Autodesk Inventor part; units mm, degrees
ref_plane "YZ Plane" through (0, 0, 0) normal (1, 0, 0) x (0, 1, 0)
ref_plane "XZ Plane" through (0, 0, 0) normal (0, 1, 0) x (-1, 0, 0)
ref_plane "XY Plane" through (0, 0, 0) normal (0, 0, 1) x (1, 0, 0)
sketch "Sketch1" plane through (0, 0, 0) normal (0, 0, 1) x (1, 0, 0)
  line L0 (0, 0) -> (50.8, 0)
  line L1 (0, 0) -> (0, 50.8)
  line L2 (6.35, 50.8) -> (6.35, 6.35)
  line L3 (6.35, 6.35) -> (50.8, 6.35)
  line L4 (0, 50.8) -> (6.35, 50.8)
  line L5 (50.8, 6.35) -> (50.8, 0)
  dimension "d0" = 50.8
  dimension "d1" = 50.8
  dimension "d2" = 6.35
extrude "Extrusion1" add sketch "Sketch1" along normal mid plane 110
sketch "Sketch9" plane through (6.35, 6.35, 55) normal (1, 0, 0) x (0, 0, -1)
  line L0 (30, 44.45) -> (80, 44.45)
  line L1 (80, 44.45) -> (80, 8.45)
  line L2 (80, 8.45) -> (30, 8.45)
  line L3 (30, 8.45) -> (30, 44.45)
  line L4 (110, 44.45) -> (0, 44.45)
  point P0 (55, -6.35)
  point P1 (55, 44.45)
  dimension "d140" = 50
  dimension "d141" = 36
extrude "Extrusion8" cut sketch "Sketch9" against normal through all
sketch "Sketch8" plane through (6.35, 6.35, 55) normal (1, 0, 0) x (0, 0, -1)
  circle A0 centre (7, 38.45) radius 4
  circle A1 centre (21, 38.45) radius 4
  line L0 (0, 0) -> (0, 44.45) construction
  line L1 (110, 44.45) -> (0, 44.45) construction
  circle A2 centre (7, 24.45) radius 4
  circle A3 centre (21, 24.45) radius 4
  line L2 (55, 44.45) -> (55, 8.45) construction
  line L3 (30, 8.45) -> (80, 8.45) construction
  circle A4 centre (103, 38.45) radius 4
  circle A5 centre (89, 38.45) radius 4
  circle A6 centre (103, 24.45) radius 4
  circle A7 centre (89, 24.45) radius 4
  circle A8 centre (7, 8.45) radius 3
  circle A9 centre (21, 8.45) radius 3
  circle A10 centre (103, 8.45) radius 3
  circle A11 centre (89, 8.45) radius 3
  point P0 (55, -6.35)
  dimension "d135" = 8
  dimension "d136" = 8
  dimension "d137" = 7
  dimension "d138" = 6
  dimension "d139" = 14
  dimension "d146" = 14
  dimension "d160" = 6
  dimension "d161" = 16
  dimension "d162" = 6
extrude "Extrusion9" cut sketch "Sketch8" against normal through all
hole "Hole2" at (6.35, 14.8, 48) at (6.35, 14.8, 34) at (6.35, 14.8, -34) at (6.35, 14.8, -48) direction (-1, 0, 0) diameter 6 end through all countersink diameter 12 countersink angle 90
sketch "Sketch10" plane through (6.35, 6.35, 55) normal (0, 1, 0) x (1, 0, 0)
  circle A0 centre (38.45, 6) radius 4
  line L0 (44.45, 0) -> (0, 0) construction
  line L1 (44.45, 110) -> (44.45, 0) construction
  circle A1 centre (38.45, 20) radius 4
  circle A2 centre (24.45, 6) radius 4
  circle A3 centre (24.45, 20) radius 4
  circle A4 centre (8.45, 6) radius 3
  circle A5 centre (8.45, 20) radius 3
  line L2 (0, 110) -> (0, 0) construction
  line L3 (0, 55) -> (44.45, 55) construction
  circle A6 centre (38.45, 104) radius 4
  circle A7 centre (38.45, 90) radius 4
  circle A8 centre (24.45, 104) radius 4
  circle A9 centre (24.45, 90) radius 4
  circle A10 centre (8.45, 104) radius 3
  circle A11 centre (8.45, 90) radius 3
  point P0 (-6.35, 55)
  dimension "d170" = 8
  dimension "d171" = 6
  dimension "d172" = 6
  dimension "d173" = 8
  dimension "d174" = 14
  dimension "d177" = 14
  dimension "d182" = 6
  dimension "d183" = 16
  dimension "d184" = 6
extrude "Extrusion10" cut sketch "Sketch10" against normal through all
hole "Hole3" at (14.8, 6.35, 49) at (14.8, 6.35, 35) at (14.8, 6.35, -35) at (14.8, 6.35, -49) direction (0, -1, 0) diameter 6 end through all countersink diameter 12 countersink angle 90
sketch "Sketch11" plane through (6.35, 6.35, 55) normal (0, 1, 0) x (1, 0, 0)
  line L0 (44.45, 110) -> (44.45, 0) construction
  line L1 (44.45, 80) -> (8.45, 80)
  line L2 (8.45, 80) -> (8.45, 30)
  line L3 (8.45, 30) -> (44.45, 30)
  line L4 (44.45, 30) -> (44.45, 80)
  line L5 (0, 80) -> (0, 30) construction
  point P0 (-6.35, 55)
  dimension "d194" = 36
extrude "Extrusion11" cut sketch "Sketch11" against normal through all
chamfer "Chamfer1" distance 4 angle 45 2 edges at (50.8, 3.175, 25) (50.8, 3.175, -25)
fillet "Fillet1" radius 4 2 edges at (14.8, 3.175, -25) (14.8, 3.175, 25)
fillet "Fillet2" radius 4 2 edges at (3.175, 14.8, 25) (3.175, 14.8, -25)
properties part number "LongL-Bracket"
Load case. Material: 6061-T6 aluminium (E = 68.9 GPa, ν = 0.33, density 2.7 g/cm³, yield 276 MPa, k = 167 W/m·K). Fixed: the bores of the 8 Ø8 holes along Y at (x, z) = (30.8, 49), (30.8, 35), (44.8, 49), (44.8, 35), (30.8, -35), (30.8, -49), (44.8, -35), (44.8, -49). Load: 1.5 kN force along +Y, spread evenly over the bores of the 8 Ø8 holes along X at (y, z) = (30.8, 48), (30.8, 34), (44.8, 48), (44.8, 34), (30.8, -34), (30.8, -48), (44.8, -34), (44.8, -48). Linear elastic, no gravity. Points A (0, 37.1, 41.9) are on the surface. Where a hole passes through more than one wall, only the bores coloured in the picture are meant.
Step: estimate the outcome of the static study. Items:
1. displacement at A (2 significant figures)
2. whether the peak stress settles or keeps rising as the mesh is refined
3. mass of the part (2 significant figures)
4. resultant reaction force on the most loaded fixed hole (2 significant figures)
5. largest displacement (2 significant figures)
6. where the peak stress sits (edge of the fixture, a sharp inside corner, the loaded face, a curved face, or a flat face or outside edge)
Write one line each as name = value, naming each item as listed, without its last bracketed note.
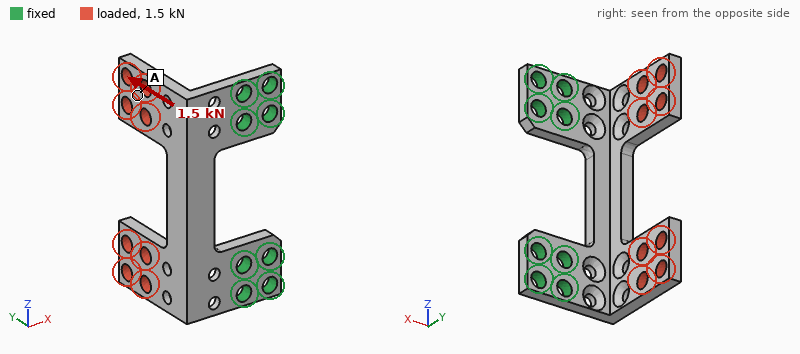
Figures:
displacement at A = 0.27 mm
whether the peak stress settles or keeps rising as the mesh is refined = keeps rising
mass of the part = 98 g
resultant reaction force on the most loaded fixed hole = 500 N
largest displacement = 0.36 mm
where the peak stress sits = a sharp inside corner
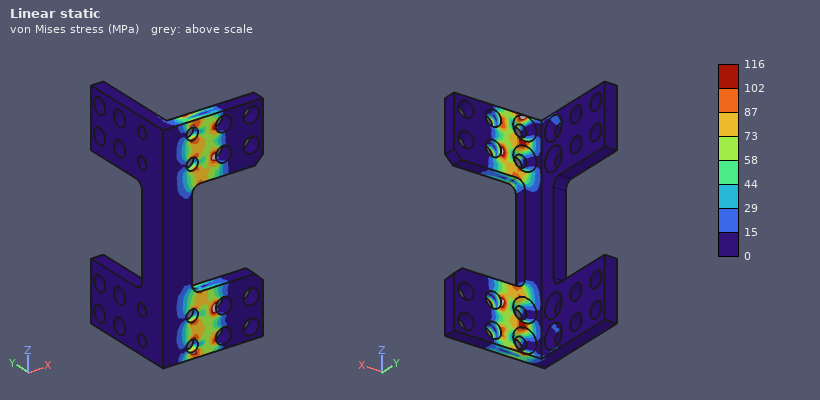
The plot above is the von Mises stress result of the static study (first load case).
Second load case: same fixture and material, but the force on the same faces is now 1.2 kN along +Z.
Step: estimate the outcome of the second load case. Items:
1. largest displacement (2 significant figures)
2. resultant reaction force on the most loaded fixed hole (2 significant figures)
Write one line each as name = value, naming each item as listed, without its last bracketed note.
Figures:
largest displacement = 0.16 mm
resultant reaction force on the most loaded fixed hole = 570 N
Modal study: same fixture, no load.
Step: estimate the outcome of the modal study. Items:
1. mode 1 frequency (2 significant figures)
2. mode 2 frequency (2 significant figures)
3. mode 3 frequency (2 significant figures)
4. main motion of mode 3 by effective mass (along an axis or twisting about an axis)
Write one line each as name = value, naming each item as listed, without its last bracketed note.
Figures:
mode 1 frequency = 1200 Hz
mode 2 frequency = 1600 Hz
mode 3 frequency = 3200 Hz
main motion of mode 3 by effective mass = along Y
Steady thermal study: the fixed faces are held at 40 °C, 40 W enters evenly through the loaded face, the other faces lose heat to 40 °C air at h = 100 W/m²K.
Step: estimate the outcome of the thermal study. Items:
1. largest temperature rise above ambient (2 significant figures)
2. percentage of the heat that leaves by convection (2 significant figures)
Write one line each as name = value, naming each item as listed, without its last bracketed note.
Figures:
largest temperature rise above ambient = 32 K
percentage of the heat that leaves by convection = 47 %
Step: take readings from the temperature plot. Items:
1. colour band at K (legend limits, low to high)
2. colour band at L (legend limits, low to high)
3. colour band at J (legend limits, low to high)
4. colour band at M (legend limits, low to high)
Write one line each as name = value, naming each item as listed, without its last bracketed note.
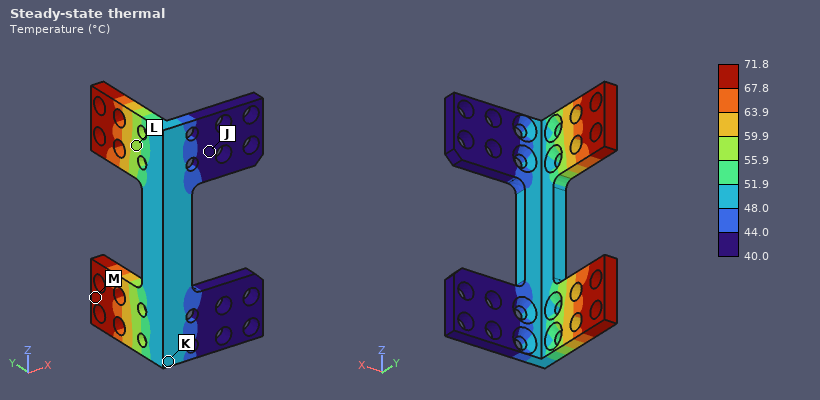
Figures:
colour band at K = 48.0 to 51.9 °C
colour band at L = 55.9 to 59.9 °C
colour band at J = 40.0 to 44.0 °C
colour band at M = 67.8 to 71.8 °C
